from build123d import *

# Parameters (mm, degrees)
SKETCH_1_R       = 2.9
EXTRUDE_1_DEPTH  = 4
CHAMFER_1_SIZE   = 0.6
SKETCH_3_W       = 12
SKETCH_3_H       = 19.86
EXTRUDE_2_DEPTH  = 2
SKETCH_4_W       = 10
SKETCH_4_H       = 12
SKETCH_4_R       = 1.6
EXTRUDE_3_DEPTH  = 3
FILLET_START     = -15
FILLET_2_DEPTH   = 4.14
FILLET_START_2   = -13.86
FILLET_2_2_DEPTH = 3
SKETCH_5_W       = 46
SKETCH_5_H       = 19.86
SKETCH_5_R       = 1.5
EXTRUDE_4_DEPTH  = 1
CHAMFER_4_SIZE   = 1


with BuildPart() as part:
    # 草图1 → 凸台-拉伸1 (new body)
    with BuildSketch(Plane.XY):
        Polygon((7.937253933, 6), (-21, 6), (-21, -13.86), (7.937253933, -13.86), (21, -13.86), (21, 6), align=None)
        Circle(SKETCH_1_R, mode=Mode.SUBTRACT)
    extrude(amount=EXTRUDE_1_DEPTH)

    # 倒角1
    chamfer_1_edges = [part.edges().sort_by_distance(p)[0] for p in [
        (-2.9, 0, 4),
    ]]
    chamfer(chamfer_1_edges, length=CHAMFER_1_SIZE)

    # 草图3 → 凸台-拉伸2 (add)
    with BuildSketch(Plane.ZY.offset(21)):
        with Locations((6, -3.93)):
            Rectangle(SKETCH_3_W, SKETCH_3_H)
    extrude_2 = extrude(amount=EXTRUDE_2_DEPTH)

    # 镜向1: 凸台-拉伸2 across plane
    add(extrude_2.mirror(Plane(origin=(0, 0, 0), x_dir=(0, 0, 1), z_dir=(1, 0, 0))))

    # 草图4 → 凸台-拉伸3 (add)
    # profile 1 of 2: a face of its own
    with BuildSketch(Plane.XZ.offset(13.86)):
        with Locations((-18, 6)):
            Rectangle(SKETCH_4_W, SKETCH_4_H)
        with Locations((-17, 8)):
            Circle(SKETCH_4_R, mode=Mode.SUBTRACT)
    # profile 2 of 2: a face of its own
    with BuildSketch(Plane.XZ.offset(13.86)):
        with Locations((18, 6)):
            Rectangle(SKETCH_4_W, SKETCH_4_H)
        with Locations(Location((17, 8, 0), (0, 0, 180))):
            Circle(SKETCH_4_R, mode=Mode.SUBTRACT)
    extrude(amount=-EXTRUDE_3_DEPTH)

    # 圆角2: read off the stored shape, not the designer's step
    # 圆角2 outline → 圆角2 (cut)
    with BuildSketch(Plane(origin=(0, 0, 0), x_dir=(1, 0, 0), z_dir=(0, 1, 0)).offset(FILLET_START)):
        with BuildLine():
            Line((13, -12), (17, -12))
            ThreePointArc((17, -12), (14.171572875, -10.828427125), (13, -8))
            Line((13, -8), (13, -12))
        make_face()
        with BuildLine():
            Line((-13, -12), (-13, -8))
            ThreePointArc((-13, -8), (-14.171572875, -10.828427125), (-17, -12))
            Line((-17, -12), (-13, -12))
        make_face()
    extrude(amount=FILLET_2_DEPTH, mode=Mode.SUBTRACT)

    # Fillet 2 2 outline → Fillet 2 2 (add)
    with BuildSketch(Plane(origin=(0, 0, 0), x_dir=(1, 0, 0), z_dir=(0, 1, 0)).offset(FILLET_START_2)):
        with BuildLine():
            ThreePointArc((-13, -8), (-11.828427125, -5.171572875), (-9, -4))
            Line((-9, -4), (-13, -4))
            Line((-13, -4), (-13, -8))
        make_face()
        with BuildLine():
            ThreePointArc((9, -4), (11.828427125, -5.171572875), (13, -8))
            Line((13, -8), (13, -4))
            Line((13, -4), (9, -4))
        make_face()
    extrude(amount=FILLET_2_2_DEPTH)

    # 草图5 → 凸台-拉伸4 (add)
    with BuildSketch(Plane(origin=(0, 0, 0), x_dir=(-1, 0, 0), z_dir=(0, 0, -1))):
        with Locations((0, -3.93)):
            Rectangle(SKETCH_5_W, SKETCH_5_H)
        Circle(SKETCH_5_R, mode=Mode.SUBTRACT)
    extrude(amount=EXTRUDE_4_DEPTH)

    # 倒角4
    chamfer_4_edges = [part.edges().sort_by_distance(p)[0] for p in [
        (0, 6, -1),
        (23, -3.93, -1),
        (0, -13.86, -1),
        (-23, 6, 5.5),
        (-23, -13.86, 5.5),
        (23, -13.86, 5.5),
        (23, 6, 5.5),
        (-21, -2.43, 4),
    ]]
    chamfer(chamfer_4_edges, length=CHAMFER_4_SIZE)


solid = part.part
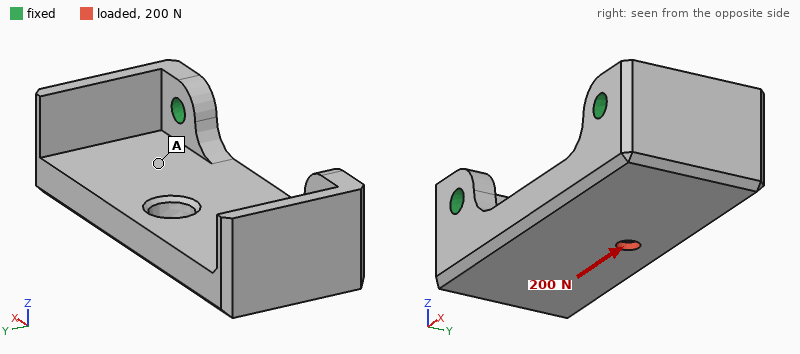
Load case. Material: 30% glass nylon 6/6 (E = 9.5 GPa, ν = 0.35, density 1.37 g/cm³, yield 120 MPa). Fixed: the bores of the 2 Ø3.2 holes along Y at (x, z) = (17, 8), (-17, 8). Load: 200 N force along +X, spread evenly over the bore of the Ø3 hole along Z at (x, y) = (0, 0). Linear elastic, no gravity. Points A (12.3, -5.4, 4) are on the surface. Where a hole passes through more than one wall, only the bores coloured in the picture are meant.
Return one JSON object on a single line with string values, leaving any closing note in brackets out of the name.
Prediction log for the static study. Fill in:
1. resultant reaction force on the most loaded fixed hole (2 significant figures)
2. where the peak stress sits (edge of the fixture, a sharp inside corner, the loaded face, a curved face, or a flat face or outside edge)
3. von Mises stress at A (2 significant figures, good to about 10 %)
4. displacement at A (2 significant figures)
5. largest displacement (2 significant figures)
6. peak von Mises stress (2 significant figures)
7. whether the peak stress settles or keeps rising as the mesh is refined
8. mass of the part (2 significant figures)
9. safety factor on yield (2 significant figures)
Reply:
{"resultant reaction force on the most loaded fixed hole": "120 N", "where the peak stress sits": "the loaded face", "von Mises stress at A": "3.5 MPa", "displacement at A": "14 µm", "largest displacement": "26 µm", "peak von Mises stress": "39 MPa", "whether the peak stress settles or keeps rising as the mesh is refined": "settles", "mass of the part": "7.3 g", "safety factor on yield": "3.1"}
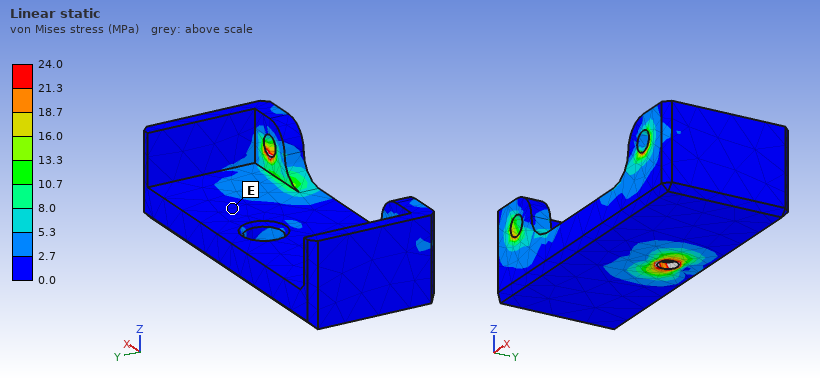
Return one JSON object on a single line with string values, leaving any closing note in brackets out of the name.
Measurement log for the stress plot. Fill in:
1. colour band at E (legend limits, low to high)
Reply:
{"colour band at E": "0.0 to 2.7 MPa"}
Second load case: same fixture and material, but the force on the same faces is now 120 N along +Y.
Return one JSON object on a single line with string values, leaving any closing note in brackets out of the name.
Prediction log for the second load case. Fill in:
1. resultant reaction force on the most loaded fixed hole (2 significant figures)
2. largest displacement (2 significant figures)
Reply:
{"resultant reaction force on the most loaded fixed hole": "62 N", "largest displacement": "95 µm"}
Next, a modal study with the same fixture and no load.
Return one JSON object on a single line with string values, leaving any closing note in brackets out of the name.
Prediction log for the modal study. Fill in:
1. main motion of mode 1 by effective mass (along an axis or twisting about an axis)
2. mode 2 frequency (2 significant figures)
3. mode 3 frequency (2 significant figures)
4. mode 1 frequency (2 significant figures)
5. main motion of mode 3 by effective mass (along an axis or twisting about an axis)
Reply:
{"main motion of mode 1 by effective mass": "along Z", "mode 2 frequency": "4500 Hz", "mode 3 frequency": "7700 Hz", "mode 1 frequency": "2300 Hz", "main motion of mode 3 by effective mass": "along X"}
